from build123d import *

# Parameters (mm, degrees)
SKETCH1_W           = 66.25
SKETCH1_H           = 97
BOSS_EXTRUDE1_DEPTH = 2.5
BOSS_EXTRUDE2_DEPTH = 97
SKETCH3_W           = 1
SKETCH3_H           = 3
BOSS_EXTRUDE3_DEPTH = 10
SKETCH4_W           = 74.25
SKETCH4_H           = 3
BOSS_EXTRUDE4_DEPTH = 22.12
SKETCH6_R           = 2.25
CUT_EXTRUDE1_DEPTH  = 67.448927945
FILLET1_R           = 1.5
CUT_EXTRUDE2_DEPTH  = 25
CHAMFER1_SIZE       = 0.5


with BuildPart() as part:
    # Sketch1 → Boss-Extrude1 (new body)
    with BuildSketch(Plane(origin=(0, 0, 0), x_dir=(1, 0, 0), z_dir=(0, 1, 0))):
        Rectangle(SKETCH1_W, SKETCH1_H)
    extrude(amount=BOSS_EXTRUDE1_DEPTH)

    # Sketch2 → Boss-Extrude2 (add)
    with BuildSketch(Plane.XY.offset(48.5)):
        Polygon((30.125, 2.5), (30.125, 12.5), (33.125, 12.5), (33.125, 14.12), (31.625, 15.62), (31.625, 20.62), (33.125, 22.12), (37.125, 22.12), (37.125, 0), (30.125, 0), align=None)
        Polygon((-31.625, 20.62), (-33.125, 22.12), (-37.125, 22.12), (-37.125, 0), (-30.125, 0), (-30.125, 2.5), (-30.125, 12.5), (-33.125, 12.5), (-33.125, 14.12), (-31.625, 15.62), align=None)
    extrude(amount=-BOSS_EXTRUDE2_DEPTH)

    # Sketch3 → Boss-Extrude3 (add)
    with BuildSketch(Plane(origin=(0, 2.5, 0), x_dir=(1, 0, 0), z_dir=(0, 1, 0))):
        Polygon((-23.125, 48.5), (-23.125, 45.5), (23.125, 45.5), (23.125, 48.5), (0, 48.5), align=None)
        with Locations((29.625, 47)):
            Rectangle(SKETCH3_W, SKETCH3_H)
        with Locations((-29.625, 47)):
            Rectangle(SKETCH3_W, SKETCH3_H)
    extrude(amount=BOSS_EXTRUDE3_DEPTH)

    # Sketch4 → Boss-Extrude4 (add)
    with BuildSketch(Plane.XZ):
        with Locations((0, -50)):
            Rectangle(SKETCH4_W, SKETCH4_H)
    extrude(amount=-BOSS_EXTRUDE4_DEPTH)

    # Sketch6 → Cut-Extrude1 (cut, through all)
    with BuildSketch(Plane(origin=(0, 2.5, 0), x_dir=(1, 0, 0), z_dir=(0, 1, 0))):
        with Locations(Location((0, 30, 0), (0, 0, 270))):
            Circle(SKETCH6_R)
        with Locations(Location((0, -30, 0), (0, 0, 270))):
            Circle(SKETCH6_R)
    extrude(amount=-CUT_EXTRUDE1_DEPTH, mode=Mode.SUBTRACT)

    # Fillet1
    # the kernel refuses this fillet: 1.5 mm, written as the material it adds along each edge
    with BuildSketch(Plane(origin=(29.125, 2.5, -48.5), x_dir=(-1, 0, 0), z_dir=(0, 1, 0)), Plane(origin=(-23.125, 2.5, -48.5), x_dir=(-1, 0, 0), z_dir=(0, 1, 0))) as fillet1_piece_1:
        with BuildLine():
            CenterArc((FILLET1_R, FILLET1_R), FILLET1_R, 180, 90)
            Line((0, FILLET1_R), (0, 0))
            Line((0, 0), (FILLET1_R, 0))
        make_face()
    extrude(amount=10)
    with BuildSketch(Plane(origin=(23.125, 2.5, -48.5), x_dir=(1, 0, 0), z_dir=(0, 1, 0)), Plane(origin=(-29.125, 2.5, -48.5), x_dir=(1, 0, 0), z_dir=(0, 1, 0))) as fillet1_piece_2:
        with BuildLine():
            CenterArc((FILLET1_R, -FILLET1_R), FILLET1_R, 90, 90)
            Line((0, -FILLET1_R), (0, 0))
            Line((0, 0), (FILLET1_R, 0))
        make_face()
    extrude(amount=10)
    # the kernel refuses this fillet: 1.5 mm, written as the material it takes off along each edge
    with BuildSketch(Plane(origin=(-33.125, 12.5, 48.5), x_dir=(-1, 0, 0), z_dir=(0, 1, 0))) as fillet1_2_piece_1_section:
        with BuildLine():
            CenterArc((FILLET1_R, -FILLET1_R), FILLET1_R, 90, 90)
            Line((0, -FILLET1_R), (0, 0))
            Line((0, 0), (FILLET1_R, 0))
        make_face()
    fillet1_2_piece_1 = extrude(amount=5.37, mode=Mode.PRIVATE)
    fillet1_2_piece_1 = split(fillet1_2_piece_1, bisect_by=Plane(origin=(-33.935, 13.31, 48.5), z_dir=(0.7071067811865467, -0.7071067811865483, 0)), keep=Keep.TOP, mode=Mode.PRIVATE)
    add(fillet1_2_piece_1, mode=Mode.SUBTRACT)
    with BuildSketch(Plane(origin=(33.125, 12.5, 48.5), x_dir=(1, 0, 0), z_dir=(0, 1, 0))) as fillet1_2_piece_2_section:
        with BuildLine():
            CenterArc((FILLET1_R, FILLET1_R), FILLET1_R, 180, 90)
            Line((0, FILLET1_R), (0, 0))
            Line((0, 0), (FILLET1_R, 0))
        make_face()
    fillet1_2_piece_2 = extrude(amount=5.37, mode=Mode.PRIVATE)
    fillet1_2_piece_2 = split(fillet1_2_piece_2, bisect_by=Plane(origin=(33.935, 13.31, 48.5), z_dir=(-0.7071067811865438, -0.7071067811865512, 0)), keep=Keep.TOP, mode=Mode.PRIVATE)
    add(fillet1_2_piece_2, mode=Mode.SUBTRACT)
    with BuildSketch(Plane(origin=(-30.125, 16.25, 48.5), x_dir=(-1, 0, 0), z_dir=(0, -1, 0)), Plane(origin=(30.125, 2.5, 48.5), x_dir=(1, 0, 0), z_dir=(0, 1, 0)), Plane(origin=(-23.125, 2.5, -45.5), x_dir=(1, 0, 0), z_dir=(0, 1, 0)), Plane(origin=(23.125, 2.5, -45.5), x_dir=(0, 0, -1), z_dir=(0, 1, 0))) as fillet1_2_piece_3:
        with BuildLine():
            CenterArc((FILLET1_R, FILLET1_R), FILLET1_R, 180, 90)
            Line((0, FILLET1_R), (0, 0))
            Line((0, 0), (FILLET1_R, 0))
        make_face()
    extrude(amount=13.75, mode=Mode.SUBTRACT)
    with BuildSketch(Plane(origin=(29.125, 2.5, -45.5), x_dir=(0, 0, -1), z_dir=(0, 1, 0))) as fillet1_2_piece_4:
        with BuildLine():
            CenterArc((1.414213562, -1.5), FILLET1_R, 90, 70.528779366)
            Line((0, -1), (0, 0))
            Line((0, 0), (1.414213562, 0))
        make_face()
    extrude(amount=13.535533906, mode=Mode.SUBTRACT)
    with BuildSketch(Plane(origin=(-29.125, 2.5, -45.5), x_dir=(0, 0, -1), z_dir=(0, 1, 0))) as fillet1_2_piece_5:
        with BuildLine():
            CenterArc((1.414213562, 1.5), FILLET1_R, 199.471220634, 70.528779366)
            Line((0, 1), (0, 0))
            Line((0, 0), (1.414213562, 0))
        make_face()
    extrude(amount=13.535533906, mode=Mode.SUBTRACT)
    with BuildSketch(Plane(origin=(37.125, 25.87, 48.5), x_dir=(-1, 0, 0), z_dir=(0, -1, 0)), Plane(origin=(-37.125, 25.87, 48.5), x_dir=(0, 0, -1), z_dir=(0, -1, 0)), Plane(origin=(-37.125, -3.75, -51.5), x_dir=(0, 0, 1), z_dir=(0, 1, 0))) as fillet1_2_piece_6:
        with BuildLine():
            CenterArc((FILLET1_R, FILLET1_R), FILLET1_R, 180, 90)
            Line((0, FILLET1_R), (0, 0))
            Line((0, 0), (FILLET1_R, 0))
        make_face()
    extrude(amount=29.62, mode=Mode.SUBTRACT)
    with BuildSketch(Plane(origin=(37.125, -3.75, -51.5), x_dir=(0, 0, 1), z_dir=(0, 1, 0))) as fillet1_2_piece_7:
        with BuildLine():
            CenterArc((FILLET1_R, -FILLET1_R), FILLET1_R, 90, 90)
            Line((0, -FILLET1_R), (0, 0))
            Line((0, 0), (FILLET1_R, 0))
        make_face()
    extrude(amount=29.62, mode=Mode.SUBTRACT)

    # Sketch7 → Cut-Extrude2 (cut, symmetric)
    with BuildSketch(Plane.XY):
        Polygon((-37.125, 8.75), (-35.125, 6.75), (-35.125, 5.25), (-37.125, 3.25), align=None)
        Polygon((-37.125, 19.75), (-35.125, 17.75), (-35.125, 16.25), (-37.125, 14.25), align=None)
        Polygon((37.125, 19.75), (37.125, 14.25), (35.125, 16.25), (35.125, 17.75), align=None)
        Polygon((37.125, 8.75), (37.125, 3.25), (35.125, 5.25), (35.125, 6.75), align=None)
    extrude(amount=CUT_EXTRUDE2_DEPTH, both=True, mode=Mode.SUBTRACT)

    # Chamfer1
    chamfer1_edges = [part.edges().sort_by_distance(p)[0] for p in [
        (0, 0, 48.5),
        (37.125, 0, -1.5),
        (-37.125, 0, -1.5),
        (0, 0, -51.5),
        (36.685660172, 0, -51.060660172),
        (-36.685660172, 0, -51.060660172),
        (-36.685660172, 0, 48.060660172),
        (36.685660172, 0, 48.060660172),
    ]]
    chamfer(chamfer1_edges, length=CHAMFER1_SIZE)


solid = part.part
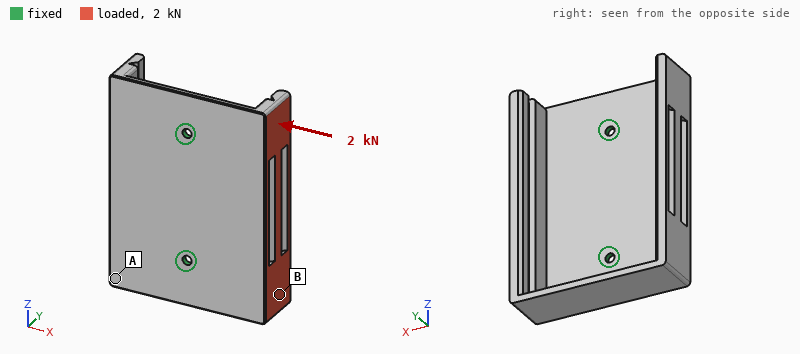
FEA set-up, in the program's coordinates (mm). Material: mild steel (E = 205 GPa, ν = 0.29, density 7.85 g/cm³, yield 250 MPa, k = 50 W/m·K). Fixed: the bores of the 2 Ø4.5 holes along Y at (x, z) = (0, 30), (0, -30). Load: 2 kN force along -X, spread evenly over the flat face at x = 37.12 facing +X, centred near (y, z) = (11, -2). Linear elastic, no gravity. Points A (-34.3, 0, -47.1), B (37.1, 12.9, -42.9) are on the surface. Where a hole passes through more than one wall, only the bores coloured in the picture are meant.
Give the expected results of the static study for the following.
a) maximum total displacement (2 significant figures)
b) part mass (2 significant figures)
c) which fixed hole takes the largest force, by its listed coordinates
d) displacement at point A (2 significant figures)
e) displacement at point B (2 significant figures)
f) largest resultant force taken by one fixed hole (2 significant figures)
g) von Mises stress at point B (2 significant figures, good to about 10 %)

0.41 mm
360 g
(0, -30)
0.26 mm
0.30 mm
1.1 kN
58 MPa
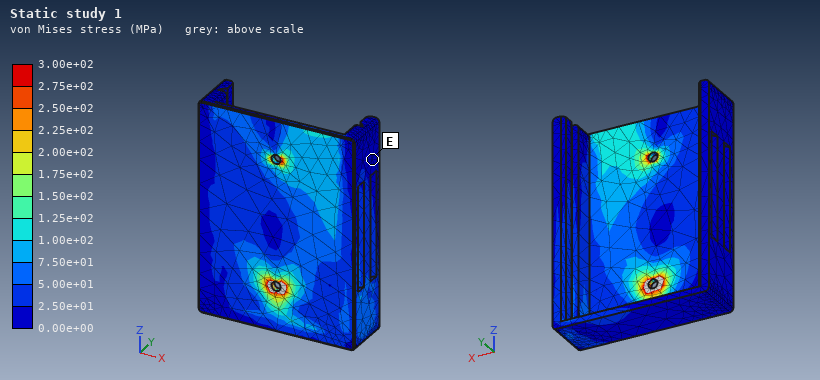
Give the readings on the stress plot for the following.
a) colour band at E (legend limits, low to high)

0.00e+00 to 2.50e+01 MPa
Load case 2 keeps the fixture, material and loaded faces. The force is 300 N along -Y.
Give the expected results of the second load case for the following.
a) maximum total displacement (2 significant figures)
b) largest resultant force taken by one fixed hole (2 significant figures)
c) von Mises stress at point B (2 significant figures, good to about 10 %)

0.19 mm
160 N
13 MPa
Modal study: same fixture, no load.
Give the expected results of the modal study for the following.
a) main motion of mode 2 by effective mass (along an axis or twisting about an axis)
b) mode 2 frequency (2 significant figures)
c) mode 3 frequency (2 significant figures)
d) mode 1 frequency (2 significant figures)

along Y
1000 Hz
1300 Hz
540 Hz
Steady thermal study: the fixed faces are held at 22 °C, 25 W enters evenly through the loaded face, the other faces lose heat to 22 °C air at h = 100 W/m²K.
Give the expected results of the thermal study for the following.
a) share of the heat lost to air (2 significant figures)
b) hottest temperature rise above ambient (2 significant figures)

84 %
31 K
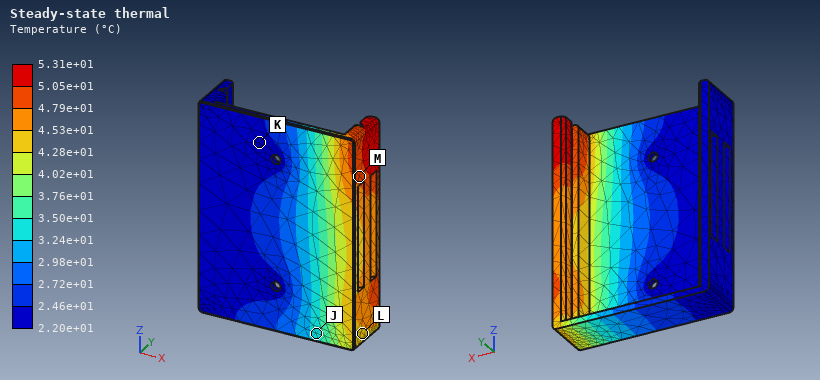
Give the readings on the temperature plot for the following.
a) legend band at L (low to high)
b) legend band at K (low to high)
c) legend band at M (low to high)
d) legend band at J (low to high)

4.28e+01 to 4.53e+01 °C
2.20e+01 to 2.46e+01 °C
4.79e+01 to 5.05e+01 °C
3.24e+01 to 3.50e+01 °C
